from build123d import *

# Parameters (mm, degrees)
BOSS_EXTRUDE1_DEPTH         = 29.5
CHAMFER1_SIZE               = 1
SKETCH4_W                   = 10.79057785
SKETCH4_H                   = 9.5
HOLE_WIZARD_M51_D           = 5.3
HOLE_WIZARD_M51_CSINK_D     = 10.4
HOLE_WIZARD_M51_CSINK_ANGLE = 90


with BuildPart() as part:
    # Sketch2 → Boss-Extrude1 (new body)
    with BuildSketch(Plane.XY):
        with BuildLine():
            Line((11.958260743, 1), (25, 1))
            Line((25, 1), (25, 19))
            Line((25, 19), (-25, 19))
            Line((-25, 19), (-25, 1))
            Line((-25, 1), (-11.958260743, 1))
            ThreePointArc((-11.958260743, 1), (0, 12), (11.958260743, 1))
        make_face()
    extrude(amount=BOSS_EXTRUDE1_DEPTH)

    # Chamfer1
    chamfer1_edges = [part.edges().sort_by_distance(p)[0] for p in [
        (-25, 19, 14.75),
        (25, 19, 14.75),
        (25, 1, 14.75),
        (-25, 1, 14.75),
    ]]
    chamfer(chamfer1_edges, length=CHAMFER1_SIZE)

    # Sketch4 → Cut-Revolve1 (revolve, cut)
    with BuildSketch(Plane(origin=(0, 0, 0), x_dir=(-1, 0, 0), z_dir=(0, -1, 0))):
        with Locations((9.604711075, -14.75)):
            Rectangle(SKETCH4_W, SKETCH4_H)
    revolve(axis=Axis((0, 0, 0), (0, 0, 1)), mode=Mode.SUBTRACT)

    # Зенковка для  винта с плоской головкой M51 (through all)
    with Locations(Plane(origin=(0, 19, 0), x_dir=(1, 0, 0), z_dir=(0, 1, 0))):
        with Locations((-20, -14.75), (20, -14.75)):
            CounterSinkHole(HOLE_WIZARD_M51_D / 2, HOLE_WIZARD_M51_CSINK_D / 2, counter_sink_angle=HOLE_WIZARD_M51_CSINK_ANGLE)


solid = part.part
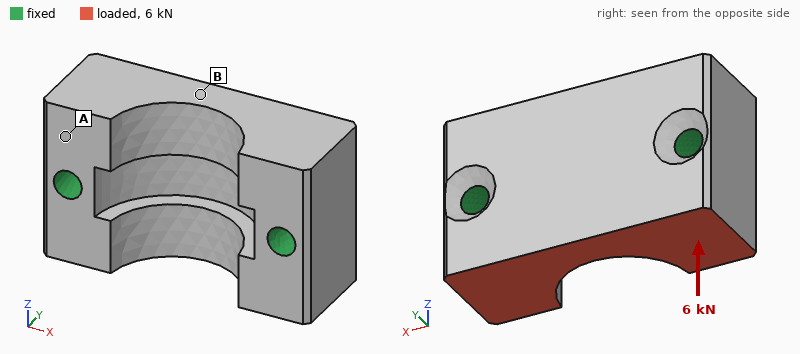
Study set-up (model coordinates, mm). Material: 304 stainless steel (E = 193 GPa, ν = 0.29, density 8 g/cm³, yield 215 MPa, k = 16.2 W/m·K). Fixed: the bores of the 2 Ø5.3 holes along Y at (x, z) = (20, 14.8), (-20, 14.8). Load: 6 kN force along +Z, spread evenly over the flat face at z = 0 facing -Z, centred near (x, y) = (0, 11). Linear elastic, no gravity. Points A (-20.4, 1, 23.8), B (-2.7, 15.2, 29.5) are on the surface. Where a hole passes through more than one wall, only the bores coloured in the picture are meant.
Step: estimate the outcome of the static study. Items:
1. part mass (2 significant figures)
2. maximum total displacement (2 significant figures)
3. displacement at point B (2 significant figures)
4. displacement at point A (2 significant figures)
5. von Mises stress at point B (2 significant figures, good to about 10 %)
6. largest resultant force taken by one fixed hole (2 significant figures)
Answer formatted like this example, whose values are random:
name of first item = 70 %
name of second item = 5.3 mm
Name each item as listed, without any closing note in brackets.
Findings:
part mass = 150 g
maximum total displacement = 2.4 µm
displacement at point B = 1.4 µm
displacement at point A = 0.38 µm
von Mises stress at point B = 9.7 MPa
largest resultant force taken by one fixed hole = 3.0 kN
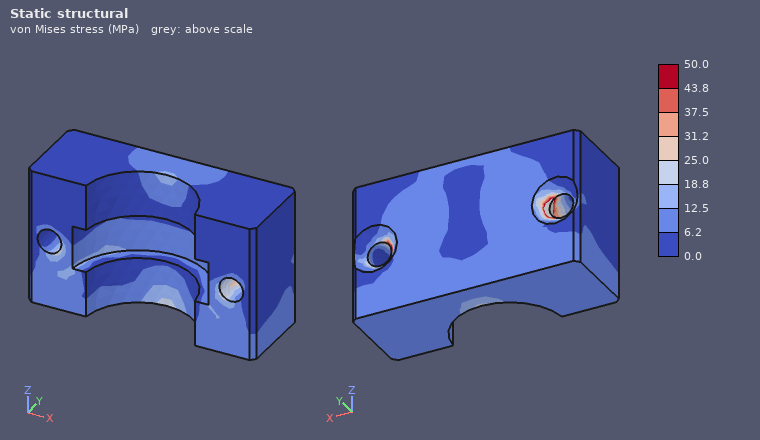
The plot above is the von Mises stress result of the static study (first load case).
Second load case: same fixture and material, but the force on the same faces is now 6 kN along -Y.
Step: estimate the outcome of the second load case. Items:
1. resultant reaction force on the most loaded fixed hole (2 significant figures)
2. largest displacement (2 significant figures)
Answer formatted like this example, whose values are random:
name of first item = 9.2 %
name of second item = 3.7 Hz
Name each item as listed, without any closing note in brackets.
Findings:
resultant reaction force on the most loaded fixed hole = 3.1 kN
largest displacement = 9.5 µm
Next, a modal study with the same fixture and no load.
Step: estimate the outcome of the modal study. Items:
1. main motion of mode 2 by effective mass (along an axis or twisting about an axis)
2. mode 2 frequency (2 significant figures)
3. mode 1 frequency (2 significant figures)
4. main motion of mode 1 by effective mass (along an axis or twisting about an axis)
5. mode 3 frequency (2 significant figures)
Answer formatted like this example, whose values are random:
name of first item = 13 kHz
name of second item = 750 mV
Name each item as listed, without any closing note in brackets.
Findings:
main motion of mode 2 by effective mass = along Y
mode 2 frequency = 26 kHz
mode 1 frequency = 23 kHz
main motion of mode 1 by effective mass = along Z
mode 3 frequency = 31 kHz
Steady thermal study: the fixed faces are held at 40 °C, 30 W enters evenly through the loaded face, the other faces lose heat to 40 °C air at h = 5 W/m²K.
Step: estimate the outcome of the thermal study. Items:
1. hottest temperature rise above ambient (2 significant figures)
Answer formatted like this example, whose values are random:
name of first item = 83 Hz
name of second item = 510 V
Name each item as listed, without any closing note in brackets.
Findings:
hottest temperature rise above ambient = 53 K
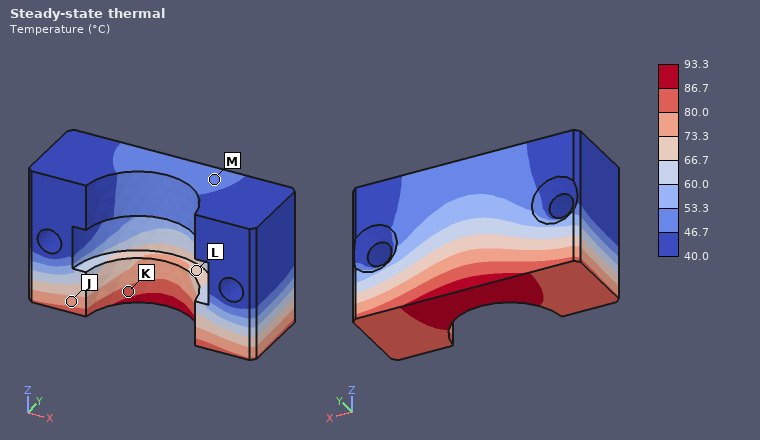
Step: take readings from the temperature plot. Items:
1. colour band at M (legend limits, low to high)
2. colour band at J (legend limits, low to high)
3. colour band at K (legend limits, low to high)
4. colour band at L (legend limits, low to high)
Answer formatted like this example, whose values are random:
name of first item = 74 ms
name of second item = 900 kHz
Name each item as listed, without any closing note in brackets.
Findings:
colour band at M = 46.7 to 53.3 °C
colour band at J = 73.3 to 80.0 °C
colour band at K = 80.0 to 86.7 °C
colour band at L = 66.7 to 73.3 °C
